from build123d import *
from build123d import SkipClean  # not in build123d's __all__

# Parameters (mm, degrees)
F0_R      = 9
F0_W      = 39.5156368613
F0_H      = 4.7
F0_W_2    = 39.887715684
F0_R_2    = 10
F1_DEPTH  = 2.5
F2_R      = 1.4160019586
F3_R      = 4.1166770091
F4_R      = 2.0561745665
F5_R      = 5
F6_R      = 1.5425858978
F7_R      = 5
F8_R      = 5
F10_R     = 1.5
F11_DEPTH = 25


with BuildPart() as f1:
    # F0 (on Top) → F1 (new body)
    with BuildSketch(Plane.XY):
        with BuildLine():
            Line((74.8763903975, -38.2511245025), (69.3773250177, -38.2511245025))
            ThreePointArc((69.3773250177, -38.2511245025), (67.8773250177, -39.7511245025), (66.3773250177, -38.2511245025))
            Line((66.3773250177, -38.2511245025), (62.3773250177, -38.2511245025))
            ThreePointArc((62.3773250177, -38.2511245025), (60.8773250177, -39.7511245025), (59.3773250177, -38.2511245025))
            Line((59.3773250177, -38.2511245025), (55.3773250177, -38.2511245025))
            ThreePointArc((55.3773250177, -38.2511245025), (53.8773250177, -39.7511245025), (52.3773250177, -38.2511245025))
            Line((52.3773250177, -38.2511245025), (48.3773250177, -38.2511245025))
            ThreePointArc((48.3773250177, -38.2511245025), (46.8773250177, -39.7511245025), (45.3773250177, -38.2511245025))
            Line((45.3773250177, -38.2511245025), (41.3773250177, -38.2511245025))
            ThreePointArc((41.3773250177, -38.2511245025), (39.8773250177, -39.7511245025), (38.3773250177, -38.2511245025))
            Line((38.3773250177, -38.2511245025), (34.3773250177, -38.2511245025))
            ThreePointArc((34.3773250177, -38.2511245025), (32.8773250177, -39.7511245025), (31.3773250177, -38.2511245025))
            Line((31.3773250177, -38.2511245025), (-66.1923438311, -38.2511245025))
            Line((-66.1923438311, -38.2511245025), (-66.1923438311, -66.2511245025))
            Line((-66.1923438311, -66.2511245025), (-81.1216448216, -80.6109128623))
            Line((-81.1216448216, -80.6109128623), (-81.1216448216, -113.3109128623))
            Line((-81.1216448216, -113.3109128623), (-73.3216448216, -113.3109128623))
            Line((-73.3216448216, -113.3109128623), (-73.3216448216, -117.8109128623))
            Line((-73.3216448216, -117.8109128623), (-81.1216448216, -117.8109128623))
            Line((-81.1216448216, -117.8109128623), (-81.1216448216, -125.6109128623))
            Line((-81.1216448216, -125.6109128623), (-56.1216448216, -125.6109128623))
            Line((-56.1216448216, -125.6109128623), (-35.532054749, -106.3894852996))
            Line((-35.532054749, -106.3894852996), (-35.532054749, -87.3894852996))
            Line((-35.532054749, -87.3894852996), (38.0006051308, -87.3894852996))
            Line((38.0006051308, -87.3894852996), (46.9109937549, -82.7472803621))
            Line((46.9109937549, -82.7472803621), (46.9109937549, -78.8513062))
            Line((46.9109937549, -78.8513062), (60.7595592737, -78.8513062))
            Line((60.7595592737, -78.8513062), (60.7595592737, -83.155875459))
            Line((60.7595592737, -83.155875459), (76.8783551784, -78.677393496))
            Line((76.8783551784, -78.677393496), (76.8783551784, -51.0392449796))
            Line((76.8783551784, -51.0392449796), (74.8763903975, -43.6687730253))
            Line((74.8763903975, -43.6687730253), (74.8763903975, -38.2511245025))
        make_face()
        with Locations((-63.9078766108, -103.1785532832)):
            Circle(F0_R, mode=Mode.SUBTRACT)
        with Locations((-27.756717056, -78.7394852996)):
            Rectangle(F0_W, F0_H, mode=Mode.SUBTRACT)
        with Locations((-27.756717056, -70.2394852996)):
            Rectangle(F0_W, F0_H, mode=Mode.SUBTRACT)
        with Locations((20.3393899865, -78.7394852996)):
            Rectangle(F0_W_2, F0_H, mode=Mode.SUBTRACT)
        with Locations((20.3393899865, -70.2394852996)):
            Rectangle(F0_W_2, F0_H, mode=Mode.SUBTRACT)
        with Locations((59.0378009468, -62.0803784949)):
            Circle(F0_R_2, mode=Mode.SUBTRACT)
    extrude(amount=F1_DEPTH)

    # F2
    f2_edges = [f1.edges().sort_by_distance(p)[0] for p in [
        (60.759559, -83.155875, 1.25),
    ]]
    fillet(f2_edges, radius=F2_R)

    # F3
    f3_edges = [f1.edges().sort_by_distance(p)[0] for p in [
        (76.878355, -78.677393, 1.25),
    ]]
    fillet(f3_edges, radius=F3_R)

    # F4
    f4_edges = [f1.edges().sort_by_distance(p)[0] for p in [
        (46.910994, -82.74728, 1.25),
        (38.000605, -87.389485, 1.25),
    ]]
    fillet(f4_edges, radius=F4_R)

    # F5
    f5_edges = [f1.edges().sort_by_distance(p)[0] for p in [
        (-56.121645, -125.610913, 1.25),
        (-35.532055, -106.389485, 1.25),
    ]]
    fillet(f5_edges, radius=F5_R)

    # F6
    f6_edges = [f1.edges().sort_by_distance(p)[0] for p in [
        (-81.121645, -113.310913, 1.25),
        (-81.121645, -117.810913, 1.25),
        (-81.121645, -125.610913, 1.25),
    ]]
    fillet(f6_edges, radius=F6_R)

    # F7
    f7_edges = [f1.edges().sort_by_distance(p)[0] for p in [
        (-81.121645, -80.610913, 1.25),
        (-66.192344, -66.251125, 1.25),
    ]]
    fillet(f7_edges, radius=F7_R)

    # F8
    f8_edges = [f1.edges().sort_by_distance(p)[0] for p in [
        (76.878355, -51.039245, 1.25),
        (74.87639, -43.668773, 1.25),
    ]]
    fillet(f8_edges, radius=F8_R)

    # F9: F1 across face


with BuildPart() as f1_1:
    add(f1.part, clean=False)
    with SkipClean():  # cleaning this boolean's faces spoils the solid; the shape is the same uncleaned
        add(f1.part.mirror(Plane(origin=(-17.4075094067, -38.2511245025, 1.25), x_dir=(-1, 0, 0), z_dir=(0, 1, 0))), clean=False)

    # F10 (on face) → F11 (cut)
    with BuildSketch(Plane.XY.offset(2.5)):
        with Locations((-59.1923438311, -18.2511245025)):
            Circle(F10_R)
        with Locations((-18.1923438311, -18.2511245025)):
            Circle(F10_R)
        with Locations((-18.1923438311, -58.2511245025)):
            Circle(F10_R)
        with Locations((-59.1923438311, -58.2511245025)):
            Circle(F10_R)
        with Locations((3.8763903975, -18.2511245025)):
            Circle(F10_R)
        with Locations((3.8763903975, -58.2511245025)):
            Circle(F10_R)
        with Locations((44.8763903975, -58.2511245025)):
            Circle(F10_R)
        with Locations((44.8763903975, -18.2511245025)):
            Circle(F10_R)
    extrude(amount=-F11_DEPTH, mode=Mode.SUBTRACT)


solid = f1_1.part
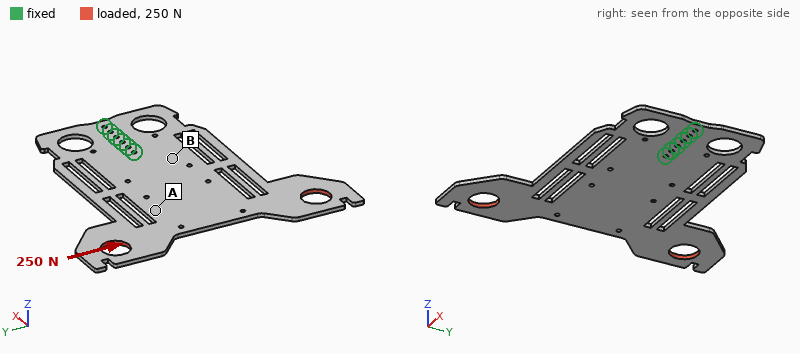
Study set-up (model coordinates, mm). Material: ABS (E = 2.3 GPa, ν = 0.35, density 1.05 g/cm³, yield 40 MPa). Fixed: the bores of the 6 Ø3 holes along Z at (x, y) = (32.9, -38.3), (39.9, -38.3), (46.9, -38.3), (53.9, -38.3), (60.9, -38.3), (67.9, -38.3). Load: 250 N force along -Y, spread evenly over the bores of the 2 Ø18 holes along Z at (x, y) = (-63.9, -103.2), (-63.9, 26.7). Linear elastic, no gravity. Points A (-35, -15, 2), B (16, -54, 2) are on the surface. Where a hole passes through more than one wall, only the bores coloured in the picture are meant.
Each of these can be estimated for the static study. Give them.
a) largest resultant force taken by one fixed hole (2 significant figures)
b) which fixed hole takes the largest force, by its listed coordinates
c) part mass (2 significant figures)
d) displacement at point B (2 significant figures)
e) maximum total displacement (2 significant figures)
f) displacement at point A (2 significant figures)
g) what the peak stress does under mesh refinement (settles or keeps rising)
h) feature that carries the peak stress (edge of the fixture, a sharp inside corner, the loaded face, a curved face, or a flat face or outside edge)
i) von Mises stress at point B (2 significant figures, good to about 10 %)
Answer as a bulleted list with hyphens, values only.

- 900 N
- (32.9, -38.3)
- 37 g
- 0.43 mm
- 2.8 mm
- 1.4 mm
- keeps rising
- edge of the fixture
- 5.1 MPa
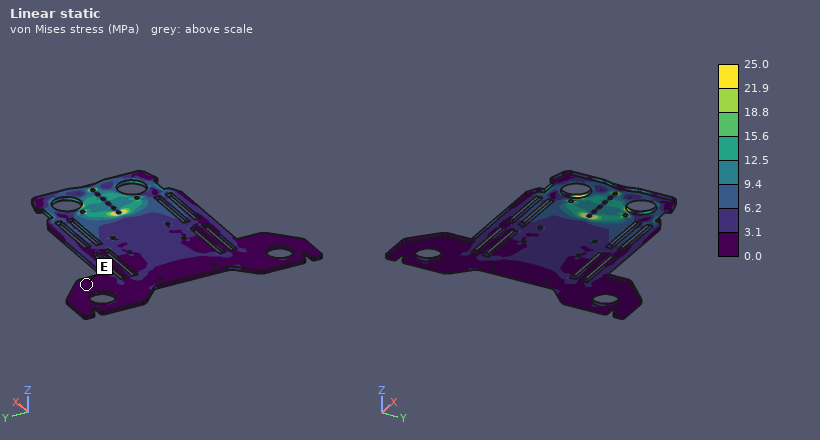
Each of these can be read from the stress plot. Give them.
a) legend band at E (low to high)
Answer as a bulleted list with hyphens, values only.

- 0.0 to 3.1 MPa
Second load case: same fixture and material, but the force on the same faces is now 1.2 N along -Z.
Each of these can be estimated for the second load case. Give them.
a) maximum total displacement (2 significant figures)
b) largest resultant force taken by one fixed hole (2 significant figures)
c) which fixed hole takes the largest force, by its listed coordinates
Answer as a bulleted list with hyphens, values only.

- 2.6 mm
- 7.1 N
- (32.9, -38.3)
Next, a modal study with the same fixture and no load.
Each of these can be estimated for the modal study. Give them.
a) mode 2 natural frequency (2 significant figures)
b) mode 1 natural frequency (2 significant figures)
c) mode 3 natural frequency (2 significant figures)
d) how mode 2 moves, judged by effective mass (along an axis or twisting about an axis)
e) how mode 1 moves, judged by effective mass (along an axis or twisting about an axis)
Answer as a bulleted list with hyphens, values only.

- 46 Hz
- 35 Hz
- 150 Hz
- twisting about X
- along Z
